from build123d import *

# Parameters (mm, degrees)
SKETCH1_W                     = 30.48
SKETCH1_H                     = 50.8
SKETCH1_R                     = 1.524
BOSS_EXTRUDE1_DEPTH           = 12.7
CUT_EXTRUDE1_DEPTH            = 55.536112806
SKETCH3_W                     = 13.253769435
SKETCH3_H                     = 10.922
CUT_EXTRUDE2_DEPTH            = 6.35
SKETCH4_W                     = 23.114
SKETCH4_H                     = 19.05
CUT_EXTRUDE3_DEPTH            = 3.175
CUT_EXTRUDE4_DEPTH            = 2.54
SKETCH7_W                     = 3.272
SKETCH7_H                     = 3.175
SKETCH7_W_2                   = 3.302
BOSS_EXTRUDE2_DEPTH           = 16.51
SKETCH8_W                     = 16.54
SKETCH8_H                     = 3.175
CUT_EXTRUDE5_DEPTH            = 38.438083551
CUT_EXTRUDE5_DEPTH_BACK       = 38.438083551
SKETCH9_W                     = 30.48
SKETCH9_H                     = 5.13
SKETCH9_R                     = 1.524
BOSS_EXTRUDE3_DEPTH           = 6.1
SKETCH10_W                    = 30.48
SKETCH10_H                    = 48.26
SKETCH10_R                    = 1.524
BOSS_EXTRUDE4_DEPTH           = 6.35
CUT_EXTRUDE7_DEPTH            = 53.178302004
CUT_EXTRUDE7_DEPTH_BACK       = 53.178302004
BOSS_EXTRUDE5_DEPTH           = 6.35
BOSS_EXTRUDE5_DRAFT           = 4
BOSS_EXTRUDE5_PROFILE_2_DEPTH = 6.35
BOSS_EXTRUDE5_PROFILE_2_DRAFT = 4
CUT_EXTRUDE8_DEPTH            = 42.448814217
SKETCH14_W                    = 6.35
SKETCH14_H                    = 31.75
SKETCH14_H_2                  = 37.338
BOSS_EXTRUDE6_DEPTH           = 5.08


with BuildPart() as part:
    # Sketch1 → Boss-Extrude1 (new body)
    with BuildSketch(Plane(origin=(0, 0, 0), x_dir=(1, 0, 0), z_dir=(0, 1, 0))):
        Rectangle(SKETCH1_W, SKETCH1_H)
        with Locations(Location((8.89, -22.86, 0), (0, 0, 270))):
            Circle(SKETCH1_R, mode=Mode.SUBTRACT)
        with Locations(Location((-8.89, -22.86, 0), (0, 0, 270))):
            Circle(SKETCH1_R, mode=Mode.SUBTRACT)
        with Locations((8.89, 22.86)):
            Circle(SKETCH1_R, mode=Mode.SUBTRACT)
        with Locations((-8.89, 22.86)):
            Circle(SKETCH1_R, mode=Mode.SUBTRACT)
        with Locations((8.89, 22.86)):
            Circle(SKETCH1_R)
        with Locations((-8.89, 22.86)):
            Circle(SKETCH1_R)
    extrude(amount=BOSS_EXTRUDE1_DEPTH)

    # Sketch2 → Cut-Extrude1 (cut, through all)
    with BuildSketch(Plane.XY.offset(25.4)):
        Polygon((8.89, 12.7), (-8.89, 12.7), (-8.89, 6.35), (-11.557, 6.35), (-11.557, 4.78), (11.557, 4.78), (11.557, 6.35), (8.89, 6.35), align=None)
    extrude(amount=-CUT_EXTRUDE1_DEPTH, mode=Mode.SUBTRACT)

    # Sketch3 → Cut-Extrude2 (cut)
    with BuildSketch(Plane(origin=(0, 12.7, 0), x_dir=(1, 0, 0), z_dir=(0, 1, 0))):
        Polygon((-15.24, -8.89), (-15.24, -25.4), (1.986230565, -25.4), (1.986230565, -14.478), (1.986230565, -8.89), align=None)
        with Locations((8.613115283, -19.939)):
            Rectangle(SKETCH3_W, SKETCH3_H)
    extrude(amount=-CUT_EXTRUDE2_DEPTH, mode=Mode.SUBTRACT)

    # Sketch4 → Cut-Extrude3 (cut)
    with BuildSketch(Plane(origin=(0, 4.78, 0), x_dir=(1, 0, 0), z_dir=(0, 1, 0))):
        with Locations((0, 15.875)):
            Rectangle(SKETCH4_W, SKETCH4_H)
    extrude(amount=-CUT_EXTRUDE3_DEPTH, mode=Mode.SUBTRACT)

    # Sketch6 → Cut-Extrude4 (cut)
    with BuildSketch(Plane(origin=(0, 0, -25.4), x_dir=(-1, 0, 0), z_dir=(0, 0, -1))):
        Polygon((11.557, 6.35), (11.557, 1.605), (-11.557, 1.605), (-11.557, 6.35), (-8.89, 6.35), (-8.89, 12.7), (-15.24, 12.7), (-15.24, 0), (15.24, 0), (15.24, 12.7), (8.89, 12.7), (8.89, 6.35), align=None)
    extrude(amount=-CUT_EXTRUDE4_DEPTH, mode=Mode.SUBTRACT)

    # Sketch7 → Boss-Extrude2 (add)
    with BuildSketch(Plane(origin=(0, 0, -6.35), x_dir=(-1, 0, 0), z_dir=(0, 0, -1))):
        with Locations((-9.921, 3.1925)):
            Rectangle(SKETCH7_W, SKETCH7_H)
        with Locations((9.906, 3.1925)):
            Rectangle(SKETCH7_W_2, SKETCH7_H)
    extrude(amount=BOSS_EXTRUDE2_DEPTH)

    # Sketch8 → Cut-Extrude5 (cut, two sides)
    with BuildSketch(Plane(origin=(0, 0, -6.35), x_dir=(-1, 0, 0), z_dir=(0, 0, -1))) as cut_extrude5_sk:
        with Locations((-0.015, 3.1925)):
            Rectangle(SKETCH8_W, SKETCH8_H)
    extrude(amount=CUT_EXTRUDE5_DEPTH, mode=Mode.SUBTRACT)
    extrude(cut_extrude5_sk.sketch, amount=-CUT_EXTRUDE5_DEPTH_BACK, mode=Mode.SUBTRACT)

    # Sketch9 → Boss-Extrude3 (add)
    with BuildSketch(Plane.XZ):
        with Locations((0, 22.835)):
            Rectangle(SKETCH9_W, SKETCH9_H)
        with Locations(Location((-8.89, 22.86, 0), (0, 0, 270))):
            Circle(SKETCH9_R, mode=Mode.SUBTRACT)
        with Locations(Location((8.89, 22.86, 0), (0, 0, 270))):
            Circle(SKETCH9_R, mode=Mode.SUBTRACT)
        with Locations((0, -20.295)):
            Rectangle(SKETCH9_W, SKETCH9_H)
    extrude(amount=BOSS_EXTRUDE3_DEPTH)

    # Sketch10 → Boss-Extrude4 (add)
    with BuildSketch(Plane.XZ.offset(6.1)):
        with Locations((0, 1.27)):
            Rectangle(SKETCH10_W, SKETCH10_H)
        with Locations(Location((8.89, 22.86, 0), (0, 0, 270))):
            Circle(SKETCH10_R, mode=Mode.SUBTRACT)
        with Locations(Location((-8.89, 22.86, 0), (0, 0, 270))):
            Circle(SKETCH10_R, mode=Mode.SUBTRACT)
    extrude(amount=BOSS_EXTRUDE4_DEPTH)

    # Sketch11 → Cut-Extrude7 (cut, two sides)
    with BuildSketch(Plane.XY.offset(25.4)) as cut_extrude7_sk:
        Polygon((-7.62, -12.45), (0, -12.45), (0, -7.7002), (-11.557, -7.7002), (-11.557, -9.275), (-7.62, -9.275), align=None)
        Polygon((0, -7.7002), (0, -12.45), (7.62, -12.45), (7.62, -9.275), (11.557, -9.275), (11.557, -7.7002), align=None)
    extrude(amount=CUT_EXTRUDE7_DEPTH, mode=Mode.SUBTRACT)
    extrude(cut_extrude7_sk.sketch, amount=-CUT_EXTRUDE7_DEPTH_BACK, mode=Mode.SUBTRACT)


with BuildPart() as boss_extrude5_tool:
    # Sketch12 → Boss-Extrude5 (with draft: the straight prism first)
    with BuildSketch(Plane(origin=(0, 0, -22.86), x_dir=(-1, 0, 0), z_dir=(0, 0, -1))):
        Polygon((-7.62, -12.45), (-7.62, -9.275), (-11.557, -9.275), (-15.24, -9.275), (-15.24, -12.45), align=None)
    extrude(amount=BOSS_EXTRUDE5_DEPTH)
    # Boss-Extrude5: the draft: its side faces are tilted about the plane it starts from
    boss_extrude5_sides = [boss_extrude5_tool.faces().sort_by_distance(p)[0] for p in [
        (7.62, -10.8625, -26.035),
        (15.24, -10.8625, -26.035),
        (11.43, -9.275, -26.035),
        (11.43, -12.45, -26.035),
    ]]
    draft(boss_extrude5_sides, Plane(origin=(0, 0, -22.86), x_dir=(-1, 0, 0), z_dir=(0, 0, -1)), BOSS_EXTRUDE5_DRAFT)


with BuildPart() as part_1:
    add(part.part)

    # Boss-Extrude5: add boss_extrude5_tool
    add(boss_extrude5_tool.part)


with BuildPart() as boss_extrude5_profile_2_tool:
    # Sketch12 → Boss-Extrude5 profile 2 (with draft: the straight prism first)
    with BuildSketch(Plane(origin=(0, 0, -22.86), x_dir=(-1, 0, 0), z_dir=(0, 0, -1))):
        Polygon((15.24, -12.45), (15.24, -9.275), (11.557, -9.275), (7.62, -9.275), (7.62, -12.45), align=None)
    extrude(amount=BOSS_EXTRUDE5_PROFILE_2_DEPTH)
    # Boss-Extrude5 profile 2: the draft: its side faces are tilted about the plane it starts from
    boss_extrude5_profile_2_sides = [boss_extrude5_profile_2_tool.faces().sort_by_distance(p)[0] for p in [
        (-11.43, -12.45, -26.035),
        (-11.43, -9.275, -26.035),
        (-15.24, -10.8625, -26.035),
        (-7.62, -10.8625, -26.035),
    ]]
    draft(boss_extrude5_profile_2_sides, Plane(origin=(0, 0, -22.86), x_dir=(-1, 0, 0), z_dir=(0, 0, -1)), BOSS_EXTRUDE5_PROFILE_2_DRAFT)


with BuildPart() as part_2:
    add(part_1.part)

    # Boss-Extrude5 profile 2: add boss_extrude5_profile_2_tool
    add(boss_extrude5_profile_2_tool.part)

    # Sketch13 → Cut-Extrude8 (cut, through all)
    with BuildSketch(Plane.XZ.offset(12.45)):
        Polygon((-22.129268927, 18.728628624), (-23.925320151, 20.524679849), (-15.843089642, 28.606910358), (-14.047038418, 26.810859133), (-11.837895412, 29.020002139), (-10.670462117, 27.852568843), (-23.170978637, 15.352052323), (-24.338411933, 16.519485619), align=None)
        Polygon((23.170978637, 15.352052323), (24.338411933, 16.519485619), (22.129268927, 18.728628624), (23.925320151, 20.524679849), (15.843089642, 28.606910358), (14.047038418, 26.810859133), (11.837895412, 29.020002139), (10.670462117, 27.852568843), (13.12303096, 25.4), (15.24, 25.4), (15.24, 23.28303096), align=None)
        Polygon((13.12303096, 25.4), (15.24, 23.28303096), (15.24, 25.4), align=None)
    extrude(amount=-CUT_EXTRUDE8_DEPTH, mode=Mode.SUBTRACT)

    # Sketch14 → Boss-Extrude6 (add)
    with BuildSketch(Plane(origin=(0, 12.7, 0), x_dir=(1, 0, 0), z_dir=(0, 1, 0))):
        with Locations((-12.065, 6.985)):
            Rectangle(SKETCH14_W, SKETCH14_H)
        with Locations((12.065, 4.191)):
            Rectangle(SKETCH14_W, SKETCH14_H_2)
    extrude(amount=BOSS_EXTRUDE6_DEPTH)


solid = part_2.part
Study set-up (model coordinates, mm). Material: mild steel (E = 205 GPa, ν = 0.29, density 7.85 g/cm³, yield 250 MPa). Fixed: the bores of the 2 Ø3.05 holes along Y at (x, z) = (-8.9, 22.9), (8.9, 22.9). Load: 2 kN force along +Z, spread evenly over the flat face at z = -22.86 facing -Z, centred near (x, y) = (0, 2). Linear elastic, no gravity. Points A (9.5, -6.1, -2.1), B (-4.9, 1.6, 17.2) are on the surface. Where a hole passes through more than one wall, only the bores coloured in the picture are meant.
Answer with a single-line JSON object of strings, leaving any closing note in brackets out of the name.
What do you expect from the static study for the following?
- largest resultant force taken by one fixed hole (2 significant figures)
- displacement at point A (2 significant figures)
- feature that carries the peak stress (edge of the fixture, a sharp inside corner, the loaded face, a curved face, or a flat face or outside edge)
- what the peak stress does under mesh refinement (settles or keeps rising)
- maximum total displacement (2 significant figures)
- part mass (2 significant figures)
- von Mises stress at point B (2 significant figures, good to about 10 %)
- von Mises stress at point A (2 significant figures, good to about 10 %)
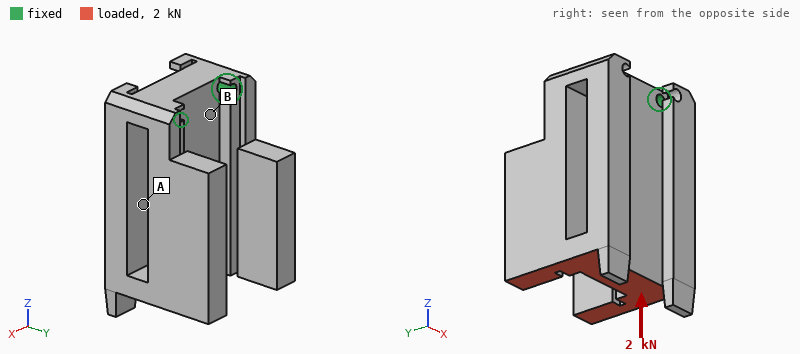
{"largest resultant force taken by one fixed hole": "1.0 kN", "displacement at point A": "8.4 µm", "feature that carries the peak stress": "edge of the fixture", "what the peak stress does under mesh refinement": "keeps rising", "maximum total displacement": "20 µm", "part mass": "130 g", "von Mises stress at point B": "18 MPa", "von Mises stress at point A": "5.3 MPa"}
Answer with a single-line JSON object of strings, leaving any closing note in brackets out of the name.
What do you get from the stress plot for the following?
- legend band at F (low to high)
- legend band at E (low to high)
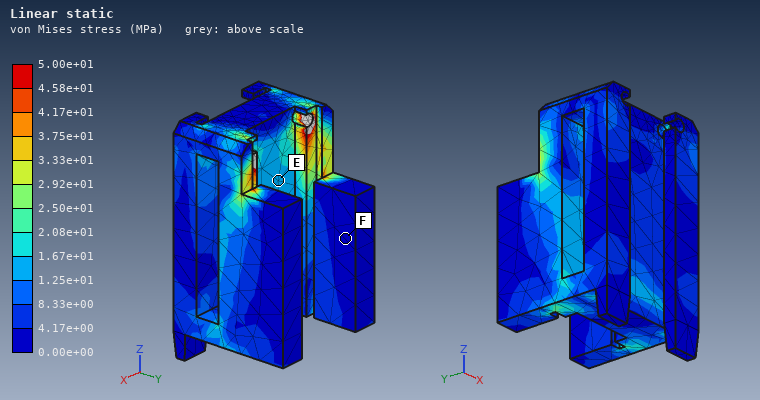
{"legend band at F": "0.00e+00 to 4.17e+00 MPa", "legend band at E": "1.25e+01 to 1.67e+01 MPa"}
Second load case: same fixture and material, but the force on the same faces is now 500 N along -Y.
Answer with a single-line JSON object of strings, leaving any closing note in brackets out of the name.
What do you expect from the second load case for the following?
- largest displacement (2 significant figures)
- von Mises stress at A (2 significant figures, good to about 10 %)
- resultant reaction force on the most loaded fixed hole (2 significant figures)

{"largest displacement": "67 µm", "von Mises stress at A": "19 MPa", "resultant reaction force on the most loaded fixed hole": "290 N"}
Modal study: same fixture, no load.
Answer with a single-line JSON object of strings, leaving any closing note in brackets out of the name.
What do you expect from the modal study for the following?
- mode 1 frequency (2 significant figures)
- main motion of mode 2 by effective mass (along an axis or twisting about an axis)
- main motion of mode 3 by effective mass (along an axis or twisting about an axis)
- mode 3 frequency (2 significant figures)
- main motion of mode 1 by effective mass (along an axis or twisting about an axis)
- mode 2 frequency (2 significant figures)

{"mode 1 frequency": "1900 Hz", "main motion of mode 2 by effective mass": "along X", "main motion of mode 3 by effective mass": "along X", "mode 3 frequency": "5200 Hz", "main motion of mode 1 by effective mass": "along Y", "mode 2 frequency": "2900 Hz"}
